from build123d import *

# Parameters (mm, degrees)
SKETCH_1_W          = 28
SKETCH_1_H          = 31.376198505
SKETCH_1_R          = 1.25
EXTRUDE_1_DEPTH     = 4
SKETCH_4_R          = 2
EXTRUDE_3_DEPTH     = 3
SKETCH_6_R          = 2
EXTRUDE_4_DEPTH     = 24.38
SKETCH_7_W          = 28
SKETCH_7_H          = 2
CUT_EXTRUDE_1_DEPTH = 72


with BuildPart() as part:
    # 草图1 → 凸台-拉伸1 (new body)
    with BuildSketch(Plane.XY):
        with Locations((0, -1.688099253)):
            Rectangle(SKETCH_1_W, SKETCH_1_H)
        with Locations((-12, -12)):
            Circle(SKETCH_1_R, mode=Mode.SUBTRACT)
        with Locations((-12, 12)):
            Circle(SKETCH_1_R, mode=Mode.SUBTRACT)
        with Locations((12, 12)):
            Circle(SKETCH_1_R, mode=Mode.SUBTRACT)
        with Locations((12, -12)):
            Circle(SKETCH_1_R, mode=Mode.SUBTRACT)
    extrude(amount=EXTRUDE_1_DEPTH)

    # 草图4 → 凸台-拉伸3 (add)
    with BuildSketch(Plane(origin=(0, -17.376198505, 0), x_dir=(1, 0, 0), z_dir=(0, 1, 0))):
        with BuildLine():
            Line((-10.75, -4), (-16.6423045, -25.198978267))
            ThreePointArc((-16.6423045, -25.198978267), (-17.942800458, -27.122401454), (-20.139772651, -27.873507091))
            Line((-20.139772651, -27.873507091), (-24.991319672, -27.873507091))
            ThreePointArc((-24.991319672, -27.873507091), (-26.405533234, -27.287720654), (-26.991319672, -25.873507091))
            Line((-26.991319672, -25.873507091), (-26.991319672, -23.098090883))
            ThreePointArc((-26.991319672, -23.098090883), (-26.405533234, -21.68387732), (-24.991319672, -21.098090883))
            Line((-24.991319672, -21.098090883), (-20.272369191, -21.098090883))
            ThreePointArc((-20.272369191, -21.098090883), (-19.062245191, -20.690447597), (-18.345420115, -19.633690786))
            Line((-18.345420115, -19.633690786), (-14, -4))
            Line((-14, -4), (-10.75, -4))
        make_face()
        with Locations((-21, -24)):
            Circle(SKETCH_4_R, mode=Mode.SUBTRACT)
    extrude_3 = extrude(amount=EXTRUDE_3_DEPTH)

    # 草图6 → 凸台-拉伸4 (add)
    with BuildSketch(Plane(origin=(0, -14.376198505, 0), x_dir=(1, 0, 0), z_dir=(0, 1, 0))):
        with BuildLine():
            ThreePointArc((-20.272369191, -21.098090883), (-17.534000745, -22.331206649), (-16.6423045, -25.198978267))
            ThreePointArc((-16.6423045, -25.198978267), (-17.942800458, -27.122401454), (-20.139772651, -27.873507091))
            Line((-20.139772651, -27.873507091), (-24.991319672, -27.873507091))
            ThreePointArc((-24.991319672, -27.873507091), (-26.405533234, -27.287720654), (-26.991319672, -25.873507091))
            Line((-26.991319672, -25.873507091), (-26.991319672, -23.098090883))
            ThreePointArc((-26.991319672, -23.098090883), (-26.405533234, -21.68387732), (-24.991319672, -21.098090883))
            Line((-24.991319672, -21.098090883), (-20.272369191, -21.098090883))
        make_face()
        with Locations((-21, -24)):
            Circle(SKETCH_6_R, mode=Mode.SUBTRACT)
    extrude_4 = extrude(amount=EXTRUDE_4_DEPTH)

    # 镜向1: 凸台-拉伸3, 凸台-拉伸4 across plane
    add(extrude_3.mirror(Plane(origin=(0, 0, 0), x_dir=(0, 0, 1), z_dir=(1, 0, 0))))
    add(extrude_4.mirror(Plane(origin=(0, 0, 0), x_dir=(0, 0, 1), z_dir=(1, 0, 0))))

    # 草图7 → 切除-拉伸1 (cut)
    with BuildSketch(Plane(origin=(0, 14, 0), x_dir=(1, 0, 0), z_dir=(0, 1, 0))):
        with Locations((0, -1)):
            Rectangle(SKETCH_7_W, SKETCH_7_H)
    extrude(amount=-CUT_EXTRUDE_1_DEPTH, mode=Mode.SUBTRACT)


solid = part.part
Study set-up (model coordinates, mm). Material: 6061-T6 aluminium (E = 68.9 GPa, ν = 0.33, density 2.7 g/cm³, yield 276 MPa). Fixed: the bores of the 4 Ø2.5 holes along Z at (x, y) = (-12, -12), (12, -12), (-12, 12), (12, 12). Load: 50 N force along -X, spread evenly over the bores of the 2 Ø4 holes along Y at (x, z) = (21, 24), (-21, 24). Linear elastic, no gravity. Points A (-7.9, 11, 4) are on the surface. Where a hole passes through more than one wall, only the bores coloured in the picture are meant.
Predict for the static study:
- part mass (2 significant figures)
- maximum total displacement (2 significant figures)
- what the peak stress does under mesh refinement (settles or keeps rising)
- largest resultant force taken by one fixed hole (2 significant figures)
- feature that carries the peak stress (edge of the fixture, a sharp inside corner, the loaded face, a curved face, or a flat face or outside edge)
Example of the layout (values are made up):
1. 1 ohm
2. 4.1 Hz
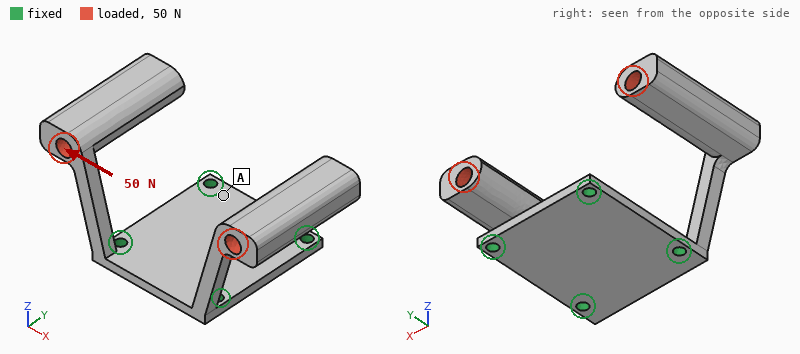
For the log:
1. 13 g
2. 0.78 mm
3. keeps rising
4. 35 N
5. edge of the fixture
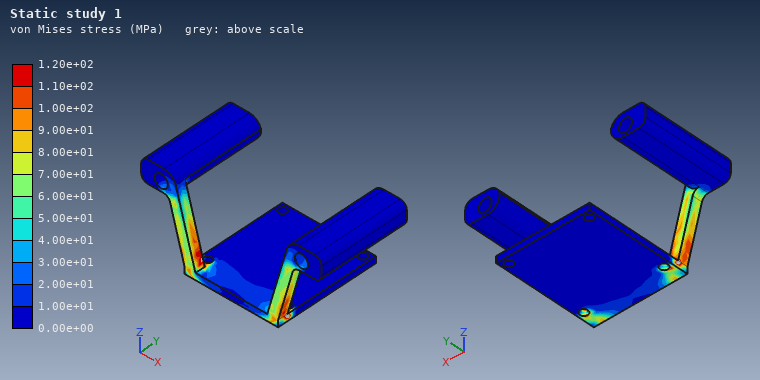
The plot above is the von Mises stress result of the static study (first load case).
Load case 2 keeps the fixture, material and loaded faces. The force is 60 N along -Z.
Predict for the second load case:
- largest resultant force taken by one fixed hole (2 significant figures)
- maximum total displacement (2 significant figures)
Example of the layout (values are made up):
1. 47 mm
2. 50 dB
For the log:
1. 27 N
2. 0.67 mm
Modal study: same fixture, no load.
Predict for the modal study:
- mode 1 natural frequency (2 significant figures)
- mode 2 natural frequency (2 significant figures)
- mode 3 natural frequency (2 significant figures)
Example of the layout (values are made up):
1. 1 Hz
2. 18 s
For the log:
1. 530 Hz
2. 530 Hz
3. 550 Hz
